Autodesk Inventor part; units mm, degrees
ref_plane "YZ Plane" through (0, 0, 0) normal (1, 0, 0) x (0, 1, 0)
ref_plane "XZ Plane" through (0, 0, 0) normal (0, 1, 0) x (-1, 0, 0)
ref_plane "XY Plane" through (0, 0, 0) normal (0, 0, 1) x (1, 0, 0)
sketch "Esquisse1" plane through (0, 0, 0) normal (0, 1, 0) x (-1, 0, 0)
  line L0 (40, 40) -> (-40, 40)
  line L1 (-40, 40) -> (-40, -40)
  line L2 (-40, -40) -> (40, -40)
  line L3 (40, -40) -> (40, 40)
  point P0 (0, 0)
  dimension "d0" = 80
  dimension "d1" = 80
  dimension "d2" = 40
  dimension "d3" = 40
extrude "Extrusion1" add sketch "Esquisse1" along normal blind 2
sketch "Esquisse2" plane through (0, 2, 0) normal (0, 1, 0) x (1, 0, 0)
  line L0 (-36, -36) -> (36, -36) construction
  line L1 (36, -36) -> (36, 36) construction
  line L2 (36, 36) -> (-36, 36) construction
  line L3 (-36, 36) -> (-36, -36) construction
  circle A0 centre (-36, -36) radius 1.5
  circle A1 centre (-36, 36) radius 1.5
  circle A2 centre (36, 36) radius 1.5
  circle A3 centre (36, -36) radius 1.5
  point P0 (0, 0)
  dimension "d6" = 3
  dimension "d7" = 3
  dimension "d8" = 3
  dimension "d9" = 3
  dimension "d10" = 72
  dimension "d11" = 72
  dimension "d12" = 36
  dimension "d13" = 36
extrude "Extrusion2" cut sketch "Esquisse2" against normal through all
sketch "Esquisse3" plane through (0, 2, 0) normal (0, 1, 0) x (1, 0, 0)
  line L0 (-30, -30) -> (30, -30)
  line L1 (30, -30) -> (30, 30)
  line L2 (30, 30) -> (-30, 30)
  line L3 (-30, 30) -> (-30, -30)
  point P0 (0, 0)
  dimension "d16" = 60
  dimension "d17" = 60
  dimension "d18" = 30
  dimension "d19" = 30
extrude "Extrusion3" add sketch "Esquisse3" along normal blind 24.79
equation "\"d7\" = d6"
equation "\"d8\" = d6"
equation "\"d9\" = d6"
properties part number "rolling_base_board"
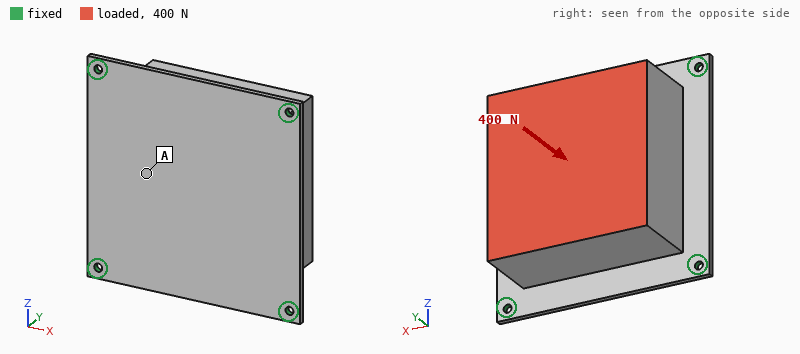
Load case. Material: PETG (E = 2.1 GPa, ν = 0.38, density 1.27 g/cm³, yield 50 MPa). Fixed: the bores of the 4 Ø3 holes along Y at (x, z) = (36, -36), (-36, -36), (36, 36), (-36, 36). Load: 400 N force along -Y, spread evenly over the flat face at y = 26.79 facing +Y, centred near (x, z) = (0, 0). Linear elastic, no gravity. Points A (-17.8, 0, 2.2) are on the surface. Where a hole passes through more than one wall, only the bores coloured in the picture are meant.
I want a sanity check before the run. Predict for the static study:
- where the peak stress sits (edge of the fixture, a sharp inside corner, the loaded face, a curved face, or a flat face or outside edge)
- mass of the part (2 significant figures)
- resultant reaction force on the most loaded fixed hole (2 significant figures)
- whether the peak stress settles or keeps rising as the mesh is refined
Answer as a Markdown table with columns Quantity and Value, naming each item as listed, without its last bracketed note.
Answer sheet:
| Quantity | Value |
|---|---|
| where the peak stress sits | edge of the fixture |
| mass of the part | 130 g |
| resultant reaction force on the most loaded fixed hole | 110 N |
| whether the peak stress settles or keeps rising as the mesh is refined | keeps rising |
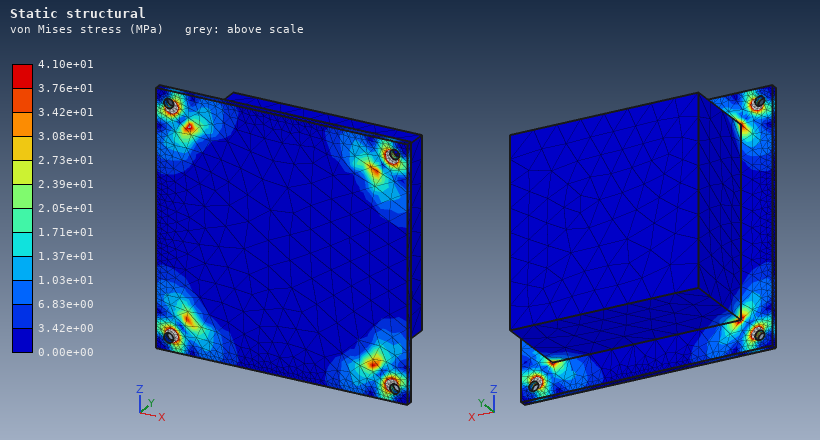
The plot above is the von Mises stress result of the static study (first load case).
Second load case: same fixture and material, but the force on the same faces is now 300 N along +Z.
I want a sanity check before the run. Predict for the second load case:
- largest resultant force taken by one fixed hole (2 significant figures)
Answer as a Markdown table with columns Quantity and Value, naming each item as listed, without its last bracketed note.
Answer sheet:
| Quantity | Value |
|---|---|
| largest resultant force taken by one fixed hole | 100 N |
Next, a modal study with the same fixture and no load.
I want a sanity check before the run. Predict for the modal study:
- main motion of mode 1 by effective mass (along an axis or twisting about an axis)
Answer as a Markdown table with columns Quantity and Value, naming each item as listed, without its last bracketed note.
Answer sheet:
| Quantity | Value |
|---|---|
| main motion of mode 1 by effective mass | along Y |
